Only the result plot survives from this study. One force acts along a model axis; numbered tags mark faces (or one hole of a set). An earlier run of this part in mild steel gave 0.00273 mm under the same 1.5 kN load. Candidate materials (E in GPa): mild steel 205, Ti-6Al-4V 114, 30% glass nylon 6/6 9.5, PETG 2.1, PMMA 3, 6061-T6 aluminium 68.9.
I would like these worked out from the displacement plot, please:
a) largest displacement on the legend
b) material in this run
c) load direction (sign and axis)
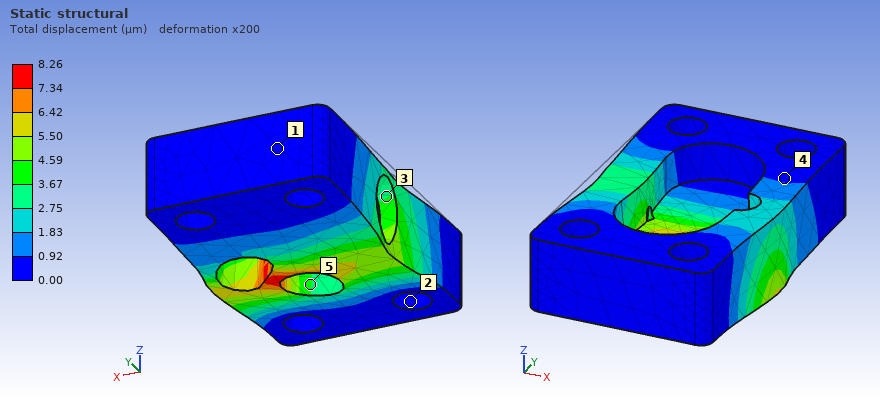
8.26 µm
6061-T6 aluminium
+X
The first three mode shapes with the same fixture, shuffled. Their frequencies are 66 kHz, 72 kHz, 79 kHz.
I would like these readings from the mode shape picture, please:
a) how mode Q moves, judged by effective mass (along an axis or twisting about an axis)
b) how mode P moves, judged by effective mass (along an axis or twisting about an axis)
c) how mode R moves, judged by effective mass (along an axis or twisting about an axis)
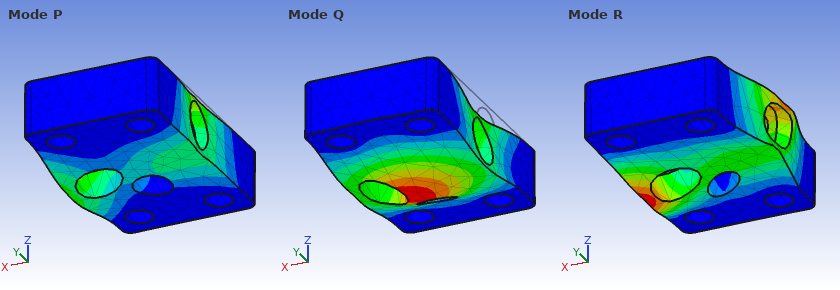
along Z
along X
along X
